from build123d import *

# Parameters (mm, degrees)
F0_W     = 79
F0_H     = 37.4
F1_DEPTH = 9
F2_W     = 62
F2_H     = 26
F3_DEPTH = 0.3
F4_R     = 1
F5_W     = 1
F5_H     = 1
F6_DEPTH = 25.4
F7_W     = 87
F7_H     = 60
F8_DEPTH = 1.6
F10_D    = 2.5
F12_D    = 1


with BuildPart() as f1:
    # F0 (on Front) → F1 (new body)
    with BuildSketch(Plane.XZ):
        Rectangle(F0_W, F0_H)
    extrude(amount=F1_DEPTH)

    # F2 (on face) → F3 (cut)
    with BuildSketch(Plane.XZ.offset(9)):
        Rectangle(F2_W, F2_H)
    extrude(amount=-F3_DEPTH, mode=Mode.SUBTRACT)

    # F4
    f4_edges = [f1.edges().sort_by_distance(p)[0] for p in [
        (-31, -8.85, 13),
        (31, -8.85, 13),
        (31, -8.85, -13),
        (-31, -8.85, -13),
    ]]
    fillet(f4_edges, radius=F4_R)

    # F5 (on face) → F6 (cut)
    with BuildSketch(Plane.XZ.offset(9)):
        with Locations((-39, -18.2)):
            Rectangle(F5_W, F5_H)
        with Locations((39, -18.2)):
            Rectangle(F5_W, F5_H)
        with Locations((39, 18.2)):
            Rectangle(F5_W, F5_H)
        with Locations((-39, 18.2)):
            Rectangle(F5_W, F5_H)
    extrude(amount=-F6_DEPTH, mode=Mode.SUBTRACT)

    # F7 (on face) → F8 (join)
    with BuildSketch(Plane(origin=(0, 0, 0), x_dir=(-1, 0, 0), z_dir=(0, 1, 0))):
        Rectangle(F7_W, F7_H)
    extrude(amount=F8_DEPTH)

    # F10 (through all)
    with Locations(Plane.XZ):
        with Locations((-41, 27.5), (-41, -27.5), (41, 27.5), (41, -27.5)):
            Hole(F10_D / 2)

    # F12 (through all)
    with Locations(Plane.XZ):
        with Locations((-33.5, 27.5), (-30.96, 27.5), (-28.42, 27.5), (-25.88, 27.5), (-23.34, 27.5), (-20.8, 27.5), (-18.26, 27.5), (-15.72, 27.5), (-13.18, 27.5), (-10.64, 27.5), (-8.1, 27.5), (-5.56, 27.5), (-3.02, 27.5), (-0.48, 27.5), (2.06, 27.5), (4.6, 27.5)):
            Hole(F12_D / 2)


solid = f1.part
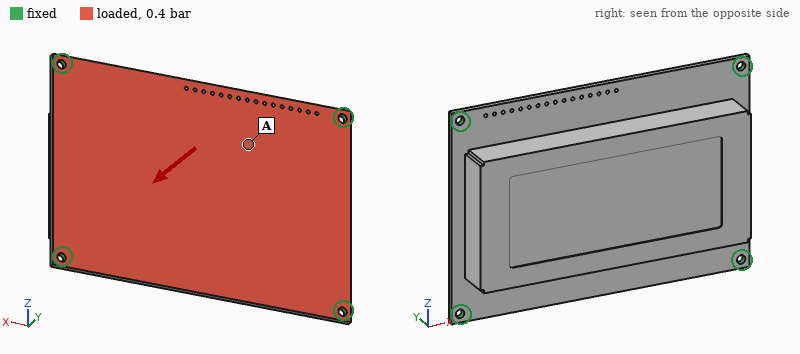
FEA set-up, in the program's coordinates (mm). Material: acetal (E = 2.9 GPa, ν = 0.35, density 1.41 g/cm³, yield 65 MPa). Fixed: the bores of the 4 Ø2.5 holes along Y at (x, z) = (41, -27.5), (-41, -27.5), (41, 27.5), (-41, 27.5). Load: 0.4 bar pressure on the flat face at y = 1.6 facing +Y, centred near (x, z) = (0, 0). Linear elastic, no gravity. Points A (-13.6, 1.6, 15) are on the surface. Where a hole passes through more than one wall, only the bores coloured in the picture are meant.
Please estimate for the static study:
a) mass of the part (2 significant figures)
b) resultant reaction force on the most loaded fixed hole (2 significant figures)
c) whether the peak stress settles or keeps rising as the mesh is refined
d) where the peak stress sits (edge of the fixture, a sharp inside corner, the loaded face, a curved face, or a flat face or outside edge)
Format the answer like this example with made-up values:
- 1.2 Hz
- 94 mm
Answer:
- 48 g
- 67 N
- keeps rising
- edge of the fixture
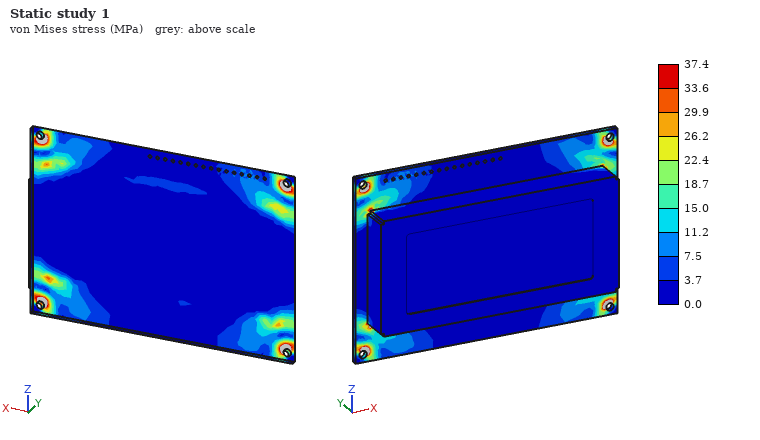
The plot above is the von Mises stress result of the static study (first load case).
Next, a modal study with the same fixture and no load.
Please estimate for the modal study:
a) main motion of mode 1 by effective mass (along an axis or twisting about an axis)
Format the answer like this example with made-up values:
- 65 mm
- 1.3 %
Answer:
- along Y
